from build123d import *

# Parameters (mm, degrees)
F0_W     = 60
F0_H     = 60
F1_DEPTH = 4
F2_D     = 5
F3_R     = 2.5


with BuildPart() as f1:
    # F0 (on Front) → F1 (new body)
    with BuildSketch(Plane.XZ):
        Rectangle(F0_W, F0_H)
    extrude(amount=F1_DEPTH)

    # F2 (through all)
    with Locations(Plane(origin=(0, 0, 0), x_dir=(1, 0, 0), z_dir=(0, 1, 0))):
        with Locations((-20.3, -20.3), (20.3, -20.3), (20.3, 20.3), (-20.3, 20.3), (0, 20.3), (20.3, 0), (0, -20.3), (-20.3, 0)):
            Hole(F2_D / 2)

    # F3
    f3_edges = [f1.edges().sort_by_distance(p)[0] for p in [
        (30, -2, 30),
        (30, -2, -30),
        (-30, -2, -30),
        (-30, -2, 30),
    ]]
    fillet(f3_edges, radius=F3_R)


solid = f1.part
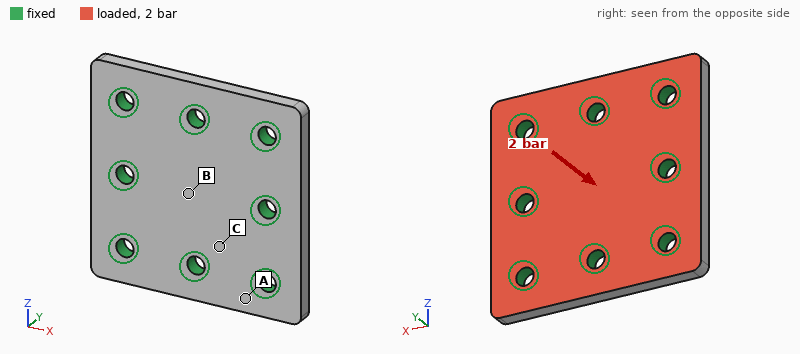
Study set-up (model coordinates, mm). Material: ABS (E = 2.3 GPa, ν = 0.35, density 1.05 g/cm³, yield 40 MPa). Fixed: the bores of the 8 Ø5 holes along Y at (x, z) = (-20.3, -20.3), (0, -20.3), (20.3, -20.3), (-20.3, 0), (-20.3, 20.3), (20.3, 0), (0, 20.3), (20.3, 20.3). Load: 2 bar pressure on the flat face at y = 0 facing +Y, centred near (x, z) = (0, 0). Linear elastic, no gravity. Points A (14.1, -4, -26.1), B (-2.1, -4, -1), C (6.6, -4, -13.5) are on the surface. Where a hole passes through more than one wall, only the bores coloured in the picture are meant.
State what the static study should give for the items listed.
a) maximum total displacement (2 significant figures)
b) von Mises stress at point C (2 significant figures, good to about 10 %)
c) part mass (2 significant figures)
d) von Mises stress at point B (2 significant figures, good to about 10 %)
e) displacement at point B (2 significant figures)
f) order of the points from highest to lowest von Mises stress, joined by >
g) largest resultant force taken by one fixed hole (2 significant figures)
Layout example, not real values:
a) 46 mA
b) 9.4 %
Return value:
a) 50 µm
b) 1.5 MPa
c) 14 g
d) 2.5 MPa
e) 49 µm
f) B > C > A
g) 98 N
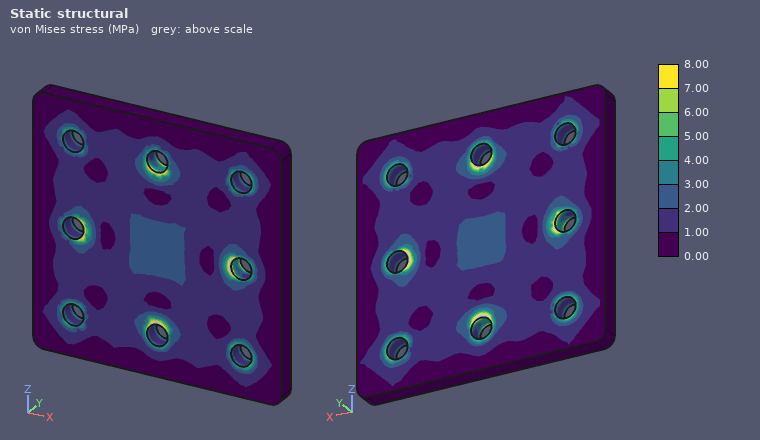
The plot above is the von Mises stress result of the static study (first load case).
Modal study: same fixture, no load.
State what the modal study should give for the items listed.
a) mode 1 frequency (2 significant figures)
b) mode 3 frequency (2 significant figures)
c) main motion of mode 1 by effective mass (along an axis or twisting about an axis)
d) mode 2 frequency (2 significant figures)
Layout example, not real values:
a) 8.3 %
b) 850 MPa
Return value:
a) 5900 Hz
b) 9700 Hz
c) along Y
d) 9600 Hz
